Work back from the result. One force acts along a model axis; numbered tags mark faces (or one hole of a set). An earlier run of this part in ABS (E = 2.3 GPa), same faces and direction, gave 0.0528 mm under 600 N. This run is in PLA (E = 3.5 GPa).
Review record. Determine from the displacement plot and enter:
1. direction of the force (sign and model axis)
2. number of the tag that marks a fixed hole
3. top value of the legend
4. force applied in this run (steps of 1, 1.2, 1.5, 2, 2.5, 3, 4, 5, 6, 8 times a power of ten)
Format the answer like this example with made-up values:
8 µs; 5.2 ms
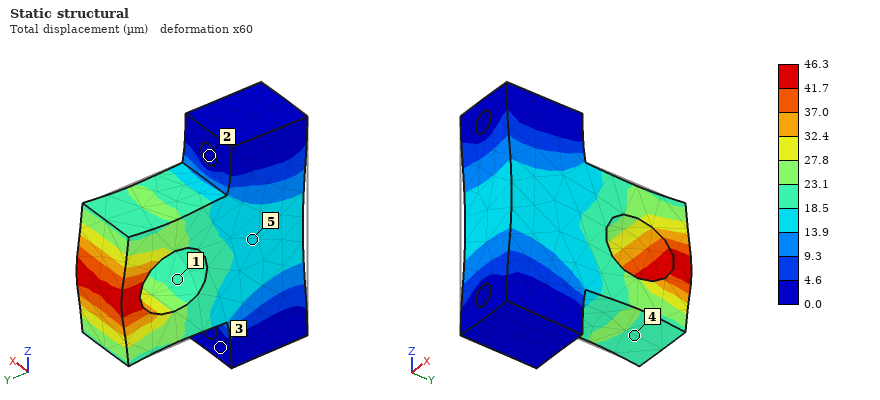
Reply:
+Y; 2; 46.3 µm; 800 N
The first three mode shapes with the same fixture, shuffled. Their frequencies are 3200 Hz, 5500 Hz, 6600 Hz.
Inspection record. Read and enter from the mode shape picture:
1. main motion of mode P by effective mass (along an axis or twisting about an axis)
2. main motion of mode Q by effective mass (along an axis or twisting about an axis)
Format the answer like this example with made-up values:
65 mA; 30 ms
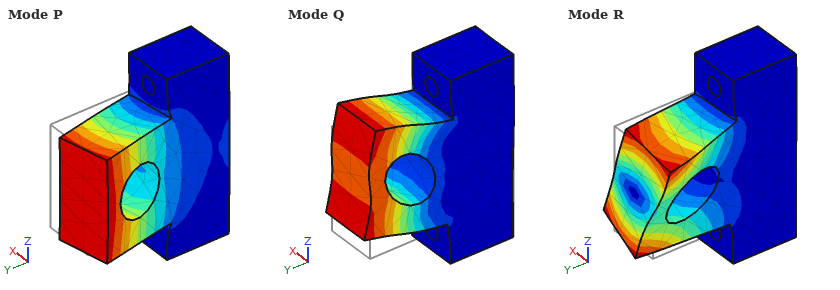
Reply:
along X; along Z
